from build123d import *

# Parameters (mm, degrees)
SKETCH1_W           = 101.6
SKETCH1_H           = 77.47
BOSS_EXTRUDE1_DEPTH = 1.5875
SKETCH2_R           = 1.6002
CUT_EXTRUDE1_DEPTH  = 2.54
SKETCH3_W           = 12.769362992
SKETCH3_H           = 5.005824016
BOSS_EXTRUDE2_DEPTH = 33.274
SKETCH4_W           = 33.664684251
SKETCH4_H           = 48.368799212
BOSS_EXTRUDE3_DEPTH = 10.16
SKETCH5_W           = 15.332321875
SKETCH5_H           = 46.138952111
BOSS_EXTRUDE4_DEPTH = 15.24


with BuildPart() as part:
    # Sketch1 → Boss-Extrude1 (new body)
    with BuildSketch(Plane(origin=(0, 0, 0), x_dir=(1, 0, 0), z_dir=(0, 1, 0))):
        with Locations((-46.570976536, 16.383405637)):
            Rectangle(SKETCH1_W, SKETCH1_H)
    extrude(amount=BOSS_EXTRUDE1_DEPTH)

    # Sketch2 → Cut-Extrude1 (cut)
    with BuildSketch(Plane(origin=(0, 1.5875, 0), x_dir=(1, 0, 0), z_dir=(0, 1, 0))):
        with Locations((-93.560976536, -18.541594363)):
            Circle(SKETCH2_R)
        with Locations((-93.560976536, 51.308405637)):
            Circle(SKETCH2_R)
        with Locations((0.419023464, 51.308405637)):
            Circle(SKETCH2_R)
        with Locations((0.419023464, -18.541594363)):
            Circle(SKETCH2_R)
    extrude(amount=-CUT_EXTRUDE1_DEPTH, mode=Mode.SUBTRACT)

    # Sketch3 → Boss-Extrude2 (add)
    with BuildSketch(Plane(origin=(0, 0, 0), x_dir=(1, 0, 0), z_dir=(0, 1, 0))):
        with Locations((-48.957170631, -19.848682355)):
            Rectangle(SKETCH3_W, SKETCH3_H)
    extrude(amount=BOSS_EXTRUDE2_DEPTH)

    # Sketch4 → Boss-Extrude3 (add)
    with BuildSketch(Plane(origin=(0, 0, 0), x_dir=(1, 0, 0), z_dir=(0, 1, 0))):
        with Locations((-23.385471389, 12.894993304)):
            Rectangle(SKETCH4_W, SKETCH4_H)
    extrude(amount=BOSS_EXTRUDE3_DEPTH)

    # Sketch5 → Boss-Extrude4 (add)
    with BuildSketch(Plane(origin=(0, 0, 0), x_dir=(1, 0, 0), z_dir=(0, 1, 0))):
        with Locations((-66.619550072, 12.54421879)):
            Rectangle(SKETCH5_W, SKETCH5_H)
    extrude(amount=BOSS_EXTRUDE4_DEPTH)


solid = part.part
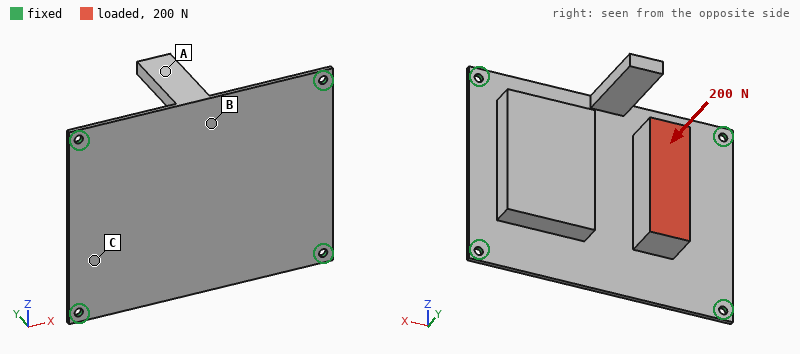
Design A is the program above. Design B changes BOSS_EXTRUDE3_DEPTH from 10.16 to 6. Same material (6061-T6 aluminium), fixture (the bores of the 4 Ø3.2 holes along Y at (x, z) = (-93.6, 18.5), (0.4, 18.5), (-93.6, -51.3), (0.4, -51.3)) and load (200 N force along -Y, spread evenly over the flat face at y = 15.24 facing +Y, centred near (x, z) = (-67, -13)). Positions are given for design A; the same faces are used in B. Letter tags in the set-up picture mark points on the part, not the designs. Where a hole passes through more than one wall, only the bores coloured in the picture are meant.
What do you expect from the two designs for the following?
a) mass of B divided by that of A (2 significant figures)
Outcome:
0.82
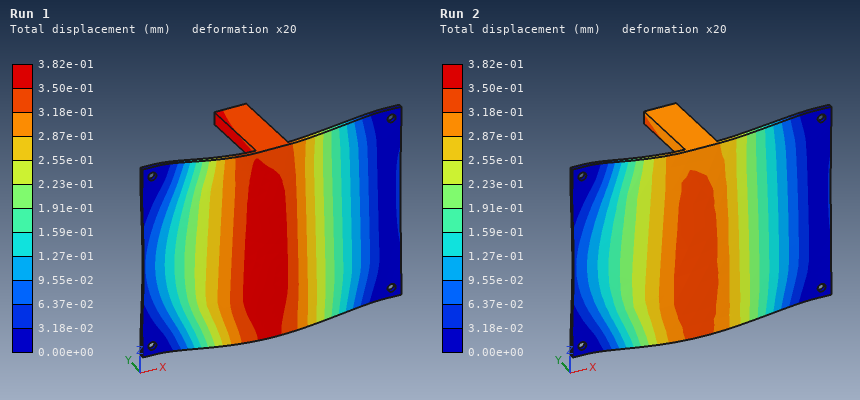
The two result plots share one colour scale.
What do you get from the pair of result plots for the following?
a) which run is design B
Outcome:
Run 2
